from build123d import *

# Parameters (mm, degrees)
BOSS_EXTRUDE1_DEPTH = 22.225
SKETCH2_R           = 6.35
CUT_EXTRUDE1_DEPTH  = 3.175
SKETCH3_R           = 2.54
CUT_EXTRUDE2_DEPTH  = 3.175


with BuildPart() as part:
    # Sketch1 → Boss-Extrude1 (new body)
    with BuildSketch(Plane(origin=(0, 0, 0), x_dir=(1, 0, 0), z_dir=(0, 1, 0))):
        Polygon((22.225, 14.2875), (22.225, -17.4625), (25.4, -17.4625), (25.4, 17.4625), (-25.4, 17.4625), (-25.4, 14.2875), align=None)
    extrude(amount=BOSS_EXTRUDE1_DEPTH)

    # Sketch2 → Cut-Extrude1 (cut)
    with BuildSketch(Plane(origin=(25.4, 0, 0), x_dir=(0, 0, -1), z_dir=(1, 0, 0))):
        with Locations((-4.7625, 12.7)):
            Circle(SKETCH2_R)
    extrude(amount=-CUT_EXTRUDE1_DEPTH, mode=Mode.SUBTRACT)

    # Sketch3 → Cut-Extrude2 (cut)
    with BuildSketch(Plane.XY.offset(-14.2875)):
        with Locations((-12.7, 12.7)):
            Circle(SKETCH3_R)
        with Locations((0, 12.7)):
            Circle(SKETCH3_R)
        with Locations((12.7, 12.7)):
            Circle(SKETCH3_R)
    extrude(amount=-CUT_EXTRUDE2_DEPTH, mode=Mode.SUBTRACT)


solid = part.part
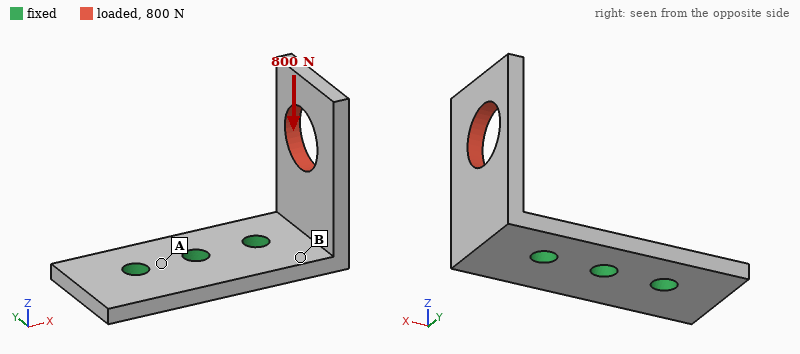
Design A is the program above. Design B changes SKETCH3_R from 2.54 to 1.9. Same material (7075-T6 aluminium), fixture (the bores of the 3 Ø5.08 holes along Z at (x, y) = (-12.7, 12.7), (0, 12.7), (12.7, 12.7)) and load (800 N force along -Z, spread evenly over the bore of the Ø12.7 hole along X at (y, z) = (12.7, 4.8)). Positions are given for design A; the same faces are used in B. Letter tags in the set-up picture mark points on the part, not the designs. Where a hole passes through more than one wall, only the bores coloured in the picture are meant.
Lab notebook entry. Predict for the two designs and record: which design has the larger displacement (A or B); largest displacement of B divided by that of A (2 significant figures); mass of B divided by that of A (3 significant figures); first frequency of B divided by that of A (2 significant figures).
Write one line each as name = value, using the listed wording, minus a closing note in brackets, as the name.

which design has the larger displacement = B
largest displacement of B divided by that of A = 1.2
mass of B divided by that of A = 1.02
first frequency of B divided by that of A = 0.98
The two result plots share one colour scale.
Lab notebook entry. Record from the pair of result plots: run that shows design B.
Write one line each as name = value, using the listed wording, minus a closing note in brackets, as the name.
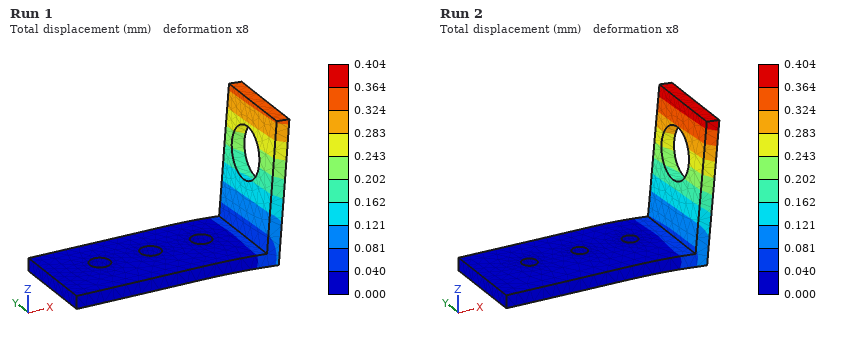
run that shows design B = Run 2
